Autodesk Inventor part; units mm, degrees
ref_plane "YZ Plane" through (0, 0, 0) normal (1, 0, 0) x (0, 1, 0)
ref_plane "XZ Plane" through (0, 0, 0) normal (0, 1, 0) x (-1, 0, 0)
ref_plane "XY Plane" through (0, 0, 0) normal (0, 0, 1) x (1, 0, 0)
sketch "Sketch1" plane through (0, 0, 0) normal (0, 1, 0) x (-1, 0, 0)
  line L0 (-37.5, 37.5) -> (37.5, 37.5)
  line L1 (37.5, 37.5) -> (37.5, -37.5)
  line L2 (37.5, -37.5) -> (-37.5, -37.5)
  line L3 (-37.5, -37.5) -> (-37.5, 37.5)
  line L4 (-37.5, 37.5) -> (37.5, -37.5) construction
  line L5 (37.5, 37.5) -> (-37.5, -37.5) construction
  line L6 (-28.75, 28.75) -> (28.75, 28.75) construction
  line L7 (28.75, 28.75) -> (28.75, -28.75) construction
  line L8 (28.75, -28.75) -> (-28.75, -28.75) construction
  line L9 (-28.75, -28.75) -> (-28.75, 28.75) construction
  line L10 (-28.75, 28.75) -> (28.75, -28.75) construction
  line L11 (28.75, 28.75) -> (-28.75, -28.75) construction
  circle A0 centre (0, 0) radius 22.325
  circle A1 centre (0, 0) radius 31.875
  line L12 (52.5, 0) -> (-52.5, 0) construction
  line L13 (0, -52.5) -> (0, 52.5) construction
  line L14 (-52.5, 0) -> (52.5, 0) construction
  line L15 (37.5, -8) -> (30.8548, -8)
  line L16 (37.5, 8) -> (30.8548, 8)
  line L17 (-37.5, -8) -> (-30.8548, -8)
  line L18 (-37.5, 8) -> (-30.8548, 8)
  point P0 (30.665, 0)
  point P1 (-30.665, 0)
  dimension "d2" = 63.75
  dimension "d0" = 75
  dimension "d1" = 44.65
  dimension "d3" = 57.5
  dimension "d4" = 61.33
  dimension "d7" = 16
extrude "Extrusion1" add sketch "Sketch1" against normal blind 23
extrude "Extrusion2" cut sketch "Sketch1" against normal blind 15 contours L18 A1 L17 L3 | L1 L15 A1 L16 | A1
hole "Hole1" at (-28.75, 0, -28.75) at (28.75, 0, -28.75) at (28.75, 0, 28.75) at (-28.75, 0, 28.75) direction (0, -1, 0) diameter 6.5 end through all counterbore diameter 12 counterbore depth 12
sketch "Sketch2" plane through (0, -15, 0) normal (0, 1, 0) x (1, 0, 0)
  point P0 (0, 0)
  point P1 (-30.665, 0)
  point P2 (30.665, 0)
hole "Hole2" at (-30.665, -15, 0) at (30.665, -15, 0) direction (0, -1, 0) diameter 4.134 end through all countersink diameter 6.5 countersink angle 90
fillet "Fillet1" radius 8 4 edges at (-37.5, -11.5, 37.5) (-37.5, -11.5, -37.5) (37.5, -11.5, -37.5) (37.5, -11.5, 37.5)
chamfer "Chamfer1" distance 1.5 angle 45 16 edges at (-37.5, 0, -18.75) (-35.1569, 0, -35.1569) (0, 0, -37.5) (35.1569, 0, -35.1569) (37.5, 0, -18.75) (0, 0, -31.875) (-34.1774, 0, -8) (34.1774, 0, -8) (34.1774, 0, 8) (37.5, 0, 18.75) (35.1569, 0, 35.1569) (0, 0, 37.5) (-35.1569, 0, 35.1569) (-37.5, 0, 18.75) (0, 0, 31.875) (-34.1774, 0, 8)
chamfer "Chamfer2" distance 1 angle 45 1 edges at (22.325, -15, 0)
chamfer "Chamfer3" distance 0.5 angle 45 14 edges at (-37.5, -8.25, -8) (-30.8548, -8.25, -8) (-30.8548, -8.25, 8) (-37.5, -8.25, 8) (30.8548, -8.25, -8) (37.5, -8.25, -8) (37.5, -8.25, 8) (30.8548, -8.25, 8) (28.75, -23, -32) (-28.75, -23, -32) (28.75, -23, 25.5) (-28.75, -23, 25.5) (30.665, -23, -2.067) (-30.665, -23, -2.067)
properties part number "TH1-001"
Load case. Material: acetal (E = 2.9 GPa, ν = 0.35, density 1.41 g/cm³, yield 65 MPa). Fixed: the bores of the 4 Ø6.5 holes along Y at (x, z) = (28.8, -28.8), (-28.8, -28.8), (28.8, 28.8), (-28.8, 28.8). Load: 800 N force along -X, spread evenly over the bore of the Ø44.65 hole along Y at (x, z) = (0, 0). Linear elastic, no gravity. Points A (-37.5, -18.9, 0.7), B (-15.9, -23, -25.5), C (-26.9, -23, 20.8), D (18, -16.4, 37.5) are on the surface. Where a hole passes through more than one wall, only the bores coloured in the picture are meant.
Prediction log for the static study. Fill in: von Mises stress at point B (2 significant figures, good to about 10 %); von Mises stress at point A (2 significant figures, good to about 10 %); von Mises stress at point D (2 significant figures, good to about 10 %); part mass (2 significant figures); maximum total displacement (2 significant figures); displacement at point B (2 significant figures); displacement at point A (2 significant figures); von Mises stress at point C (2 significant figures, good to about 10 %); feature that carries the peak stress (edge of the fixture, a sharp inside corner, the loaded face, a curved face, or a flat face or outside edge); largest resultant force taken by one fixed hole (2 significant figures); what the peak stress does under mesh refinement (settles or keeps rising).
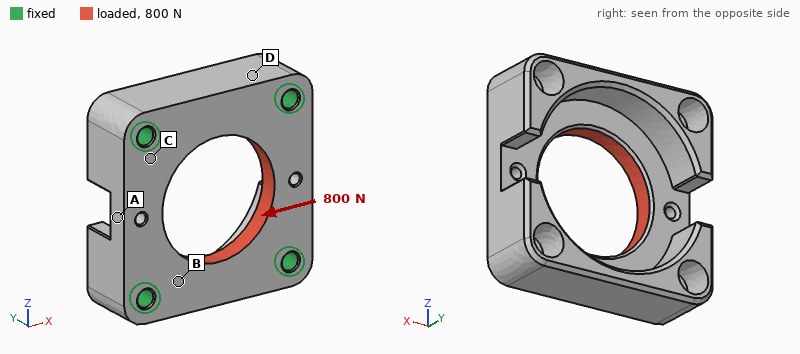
1.0 MPa
1.6 MPa
0.62 MPa
81 g
26 µm
5.1 µm
20 µm
1.3 MPa
edge of the fixture
210 N
keeps rising
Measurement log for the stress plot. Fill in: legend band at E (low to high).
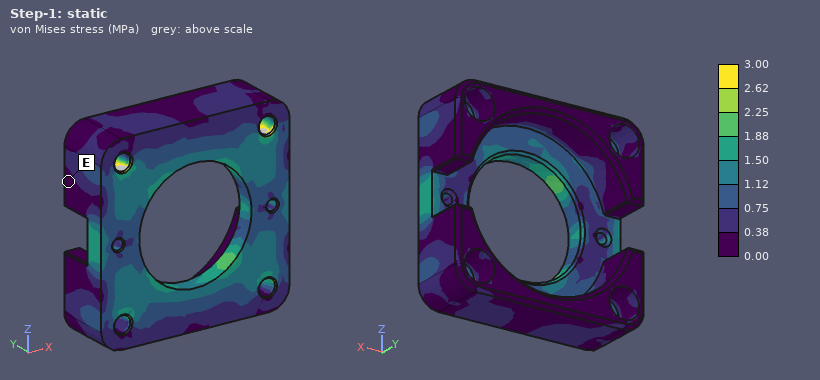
0.00 to 0.38 MPa
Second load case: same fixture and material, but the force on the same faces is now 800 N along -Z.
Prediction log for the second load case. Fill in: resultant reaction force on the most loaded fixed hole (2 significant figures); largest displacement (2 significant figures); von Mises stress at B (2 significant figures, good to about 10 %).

200 N
26 µm
1.3 MPa
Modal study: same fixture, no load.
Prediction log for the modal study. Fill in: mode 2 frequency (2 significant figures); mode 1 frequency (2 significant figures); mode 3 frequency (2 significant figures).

3800 Hz
3400 Hz
4000 Hz
